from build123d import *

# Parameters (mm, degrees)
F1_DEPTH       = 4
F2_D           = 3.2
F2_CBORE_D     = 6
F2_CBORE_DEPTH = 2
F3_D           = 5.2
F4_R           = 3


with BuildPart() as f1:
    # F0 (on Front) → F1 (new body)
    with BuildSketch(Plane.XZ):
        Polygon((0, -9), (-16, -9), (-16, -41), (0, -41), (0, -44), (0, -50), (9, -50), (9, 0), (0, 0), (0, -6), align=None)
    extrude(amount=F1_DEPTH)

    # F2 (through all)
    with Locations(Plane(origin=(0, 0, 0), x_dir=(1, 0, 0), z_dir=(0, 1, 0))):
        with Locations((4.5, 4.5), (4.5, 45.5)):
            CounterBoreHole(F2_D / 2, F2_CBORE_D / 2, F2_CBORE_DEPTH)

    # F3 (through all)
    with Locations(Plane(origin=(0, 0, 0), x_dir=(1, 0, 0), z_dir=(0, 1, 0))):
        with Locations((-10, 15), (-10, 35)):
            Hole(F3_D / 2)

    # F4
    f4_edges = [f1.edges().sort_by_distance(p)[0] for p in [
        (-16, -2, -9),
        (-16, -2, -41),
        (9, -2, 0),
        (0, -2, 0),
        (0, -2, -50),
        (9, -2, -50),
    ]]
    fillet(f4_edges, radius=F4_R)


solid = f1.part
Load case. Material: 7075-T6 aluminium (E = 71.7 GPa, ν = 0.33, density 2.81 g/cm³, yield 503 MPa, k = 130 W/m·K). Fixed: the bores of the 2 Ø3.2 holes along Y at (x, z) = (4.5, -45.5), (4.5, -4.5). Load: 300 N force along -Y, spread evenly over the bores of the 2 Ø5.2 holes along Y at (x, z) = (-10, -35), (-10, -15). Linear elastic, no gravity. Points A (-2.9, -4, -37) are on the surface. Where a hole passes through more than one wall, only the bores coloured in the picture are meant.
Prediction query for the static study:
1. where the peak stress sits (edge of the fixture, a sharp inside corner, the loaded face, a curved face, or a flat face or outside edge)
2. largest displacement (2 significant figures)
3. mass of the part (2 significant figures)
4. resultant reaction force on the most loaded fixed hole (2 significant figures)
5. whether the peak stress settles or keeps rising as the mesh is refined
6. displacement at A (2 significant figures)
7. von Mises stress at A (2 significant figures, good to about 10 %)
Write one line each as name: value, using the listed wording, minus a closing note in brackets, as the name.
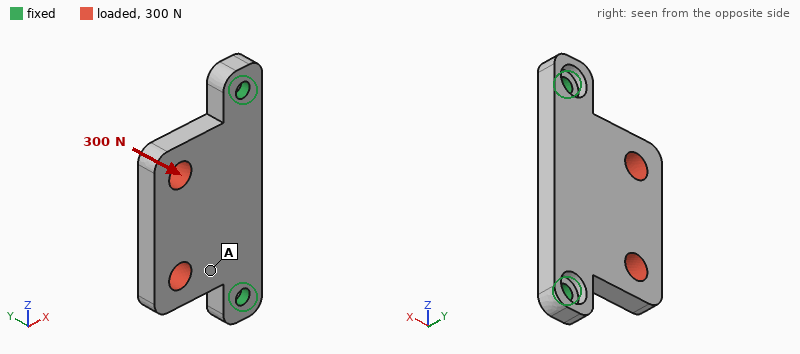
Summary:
where the peak stress sits: edge of the fixture
largest displacement: 0.19 mm
mass of the part: 9.8 g
resultant reaction force on the most loaded fixed hole: 220 N
whether the peak stress settles or keeps rising as the mesh is refined: keeps rising
displacement at A: 0.064 mm
von Mises stress at A: 39 MPa
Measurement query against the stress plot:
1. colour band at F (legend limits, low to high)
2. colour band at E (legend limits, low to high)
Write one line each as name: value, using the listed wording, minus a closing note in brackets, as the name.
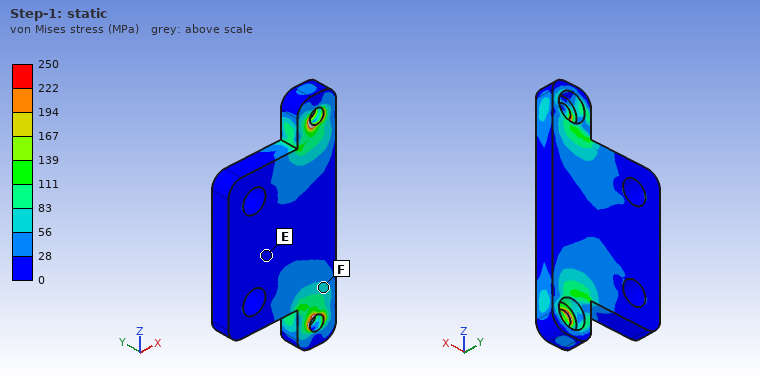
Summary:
colour band at F: 56 to 83 MPa
colour band at E: 0 to 28 MPa
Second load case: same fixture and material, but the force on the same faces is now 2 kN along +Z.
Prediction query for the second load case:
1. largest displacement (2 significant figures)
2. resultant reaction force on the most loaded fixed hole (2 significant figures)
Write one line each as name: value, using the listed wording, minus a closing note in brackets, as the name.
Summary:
largest displacement: 30 µm
resultant reaction force on the most loaded fixed hole: 1.3 kN
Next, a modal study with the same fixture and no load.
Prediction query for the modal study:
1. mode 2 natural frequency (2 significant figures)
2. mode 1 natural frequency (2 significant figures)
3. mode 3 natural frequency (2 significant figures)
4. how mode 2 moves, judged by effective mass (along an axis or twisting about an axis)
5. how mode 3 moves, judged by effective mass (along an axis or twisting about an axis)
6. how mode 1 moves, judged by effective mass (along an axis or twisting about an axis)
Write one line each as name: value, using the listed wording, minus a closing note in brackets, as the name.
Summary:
mode 2 natural frequency: 11 kHz
mode 1 natural frequency: 3600 Hz
mode 3 natural frequency: 11 kHz
how mode 2 moves, judged by effective mass: along Y
how mode 3 moves, judged by effective mass: twisting about X
how mode 1 moves, judged by effective mass: along Y
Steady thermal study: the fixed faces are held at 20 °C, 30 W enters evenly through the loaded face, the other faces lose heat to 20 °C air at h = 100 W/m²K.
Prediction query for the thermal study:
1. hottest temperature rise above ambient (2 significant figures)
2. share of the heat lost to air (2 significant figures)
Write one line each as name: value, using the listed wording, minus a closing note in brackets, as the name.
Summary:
hottest temperature rise above ambient: 51 K
share of the heat lost to air: 23 %
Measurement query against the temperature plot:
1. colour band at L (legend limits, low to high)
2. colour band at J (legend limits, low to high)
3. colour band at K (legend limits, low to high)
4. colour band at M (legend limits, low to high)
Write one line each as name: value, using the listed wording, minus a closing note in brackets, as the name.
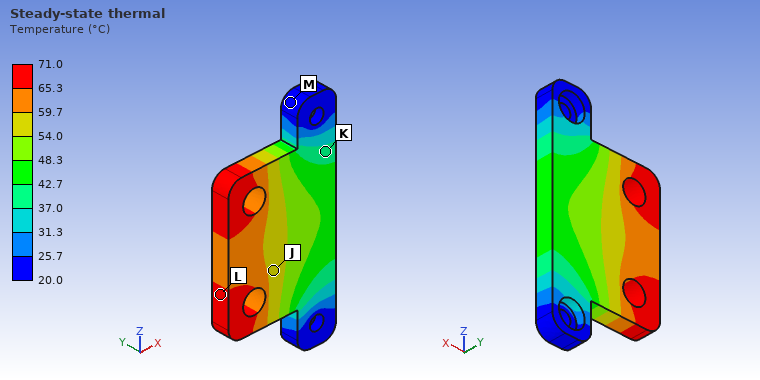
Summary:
colour band at L: 65.3 to 71.0 °C
colour band at J: 54.0 to 59.7 °C
colour band at K: 37.0 to 42.7 °C
colour band at M: 20.0 to 25.7 °C
